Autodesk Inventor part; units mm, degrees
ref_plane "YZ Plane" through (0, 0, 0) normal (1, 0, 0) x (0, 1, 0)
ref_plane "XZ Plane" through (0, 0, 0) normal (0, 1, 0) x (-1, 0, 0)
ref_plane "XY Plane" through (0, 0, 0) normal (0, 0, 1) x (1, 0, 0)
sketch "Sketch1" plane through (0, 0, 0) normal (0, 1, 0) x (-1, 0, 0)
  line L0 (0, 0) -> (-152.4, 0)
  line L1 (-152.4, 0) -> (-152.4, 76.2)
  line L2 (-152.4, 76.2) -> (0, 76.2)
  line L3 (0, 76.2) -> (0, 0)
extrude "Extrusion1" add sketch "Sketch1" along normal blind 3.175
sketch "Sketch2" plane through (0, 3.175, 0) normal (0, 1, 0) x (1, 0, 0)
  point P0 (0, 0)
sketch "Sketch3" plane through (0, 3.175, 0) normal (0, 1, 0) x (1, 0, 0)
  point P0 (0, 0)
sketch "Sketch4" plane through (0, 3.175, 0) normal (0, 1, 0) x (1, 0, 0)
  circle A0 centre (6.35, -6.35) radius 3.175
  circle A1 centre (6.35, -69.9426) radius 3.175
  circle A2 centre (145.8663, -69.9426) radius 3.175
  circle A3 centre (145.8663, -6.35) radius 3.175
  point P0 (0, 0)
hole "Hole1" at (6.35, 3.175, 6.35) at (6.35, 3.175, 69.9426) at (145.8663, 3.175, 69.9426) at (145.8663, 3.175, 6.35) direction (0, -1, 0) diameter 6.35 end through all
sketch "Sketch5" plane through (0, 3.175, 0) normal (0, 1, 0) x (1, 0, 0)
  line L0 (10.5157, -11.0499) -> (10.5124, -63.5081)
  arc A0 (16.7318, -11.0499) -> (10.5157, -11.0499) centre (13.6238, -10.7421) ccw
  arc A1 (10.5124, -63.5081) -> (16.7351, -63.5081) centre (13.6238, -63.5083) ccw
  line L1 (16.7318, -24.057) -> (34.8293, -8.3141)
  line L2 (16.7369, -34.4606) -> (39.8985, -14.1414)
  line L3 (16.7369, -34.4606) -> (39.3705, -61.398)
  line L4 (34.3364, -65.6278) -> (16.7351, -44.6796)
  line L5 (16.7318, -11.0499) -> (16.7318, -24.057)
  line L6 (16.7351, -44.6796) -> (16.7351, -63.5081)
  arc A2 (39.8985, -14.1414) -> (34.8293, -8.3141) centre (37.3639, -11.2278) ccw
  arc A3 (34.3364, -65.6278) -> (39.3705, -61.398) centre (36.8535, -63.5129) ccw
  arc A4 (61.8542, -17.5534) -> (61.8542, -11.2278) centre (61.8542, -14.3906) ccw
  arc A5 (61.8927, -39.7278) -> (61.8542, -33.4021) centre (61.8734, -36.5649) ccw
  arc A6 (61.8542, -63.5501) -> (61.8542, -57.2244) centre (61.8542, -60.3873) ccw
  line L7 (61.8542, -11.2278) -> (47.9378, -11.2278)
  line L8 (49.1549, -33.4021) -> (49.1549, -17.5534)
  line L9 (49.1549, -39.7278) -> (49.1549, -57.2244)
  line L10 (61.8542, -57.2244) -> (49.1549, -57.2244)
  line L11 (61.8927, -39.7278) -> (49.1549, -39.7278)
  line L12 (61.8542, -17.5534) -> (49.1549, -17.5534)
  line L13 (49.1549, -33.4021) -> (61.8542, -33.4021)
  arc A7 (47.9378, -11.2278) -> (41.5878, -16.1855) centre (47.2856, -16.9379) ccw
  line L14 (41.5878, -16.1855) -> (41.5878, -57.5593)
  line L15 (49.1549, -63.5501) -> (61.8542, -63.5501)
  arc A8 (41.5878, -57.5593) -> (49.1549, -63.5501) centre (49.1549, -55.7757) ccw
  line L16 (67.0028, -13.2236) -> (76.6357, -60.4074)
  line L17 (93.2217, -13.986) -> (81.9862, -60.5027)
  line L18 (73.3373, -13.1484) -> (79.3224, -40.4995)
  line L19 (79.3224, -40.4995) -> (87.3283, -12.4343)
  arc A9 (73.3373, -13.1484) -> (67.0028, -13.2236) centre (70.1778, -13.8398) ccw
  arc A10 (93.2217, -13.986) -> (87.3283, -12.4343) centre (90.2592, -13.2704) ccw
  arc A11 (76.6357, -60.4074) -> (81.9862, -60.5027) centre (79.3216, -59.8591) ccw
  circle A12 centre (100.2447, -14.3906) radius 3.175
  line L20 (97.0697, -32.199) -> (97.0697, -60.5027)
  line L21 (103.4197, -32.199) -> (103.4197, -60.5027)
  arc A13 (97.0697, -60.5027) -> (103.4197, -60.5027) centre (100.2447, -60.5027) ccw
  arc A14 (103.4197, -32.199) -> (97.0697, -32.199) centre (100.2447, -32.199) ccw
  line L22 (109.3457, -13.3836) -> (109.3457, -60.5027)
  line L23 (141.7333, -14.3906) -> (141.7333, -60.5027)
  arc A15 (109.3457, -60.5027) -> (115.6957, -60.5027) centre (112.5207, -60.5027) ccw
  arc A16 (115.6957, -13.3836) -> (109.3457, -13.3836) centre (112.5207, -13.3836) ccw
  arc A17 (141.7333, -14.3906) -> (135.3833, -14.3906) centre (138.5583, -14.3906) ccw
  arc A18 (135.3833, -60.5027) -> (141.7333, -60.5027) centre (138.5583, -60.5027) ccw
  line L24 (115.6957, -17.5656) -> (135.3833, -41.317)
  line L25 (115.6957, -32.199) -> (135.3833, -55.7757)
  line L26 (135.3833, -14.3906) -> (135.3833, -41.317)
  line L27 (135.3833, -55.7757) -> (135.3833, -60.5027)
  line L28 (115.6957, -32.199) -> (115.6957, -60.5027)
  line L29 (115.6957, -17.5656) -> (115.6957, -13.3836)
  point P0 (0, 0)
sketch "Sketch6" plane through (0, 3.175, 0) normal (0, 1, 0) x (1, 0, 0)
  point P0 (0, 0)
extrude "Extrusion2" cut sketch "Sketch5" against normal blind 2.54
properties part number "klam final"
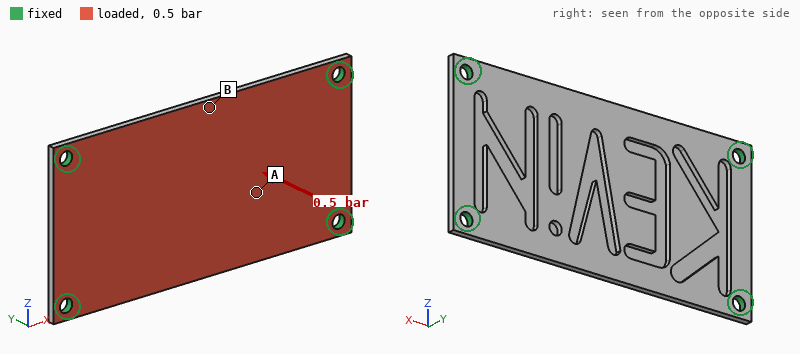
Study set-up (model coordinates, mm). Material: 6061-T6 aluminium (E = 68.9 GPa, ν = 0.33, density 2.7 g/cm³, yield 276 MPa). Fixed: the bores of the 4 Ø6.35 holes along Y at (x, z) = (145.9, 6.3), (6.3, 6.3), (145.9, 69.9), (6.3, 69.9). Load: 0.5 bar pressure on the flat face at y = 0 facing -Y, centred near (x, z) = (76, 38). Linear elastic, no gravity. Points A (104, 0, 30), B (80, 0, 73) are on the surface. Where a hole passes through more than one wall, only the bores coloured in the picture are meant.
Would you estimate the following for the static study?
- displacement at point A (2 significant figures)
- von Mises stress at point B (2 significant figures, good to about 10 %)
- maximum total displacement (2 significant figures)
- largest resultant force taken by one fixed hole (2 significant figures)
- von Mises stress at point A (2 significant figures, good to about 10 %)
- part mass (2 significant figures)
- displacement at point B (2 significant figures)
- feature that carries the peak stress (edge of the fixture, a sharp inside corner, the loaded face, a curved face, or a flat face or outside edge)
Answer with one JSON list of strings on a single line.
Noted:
["0.39 mm", "46 MPa", "0.57 mm", "240 N", "13 MPa", "76 g", "0.49 mm", "a curved face"]
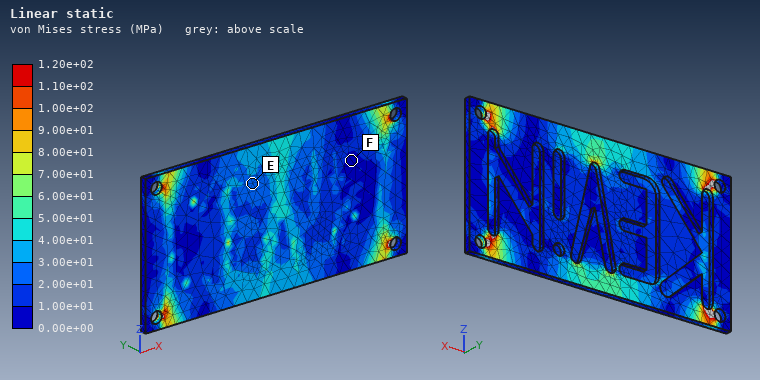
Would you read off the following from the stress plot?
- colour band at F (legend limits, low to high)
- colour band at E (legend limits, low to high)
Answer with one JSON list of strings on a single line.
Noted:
["0.00e+00 to 1.00e+01 MPa", "2.00e+01 to 3.00e+01 MPa"]
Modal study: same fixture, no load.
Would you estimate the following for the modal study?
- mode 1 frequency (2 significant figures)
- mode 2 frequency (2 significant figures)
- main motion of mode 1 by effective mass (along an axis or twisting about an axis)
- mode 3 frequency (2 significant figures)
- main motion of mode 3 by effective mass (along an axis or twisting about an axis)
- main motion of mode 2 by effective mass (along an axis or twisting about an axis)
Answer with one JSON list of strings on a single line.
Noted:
["690 Hz", "1100 Hz", "along Y", "1800 Hz", "twisting about Z", "twisting about X"]
